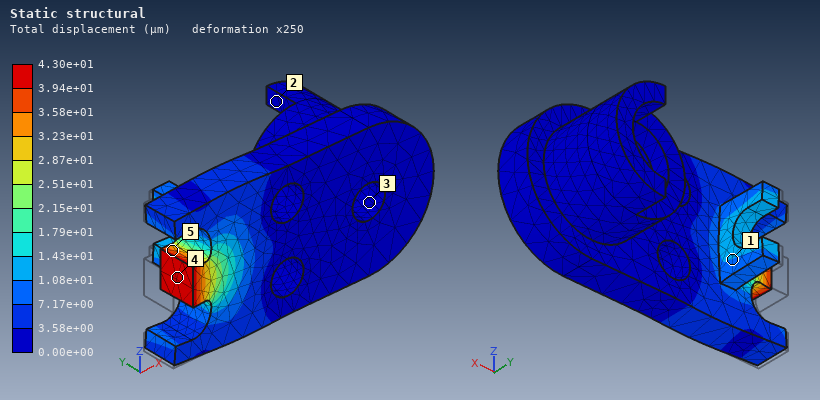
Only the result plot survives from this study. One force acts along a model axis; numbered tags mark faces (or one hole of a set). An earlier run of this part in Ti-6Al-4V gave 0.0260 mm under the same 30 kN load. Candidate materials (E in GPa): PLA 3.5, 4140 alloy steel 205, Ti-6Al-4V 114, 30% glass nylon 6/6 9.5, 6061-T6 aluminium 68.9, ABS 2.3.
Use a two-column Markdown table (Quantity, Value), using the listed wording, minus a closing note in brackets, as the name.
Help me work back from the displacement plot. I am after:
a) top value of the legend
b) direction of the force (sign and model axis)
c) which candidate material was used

| Quantity | Value |
|---|---|
| top value of the legend | 4.30e+01 µm |
| direction of the force | +X |
| which candidate material was used | 6061-T6 aluminium |
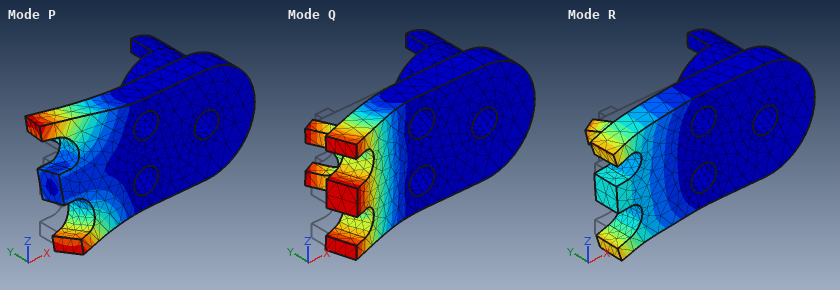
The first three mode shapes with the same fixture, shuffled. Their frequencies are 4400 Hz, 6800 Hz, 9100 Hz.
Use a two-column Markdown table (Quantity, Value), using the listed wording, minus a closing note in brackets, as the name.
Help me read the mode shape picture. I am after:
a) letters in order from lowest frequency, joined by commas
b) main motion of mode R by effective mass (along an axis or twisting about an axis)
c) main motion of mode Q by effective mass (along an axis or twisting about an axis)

| Quantity | Value |
|---|---|
| letters in order from lowest frequency, joined by commas | Q, P, R |
| main motion of mode R by effective mass | along Z |
| main motion of mode Q by effective mass | along Y |
